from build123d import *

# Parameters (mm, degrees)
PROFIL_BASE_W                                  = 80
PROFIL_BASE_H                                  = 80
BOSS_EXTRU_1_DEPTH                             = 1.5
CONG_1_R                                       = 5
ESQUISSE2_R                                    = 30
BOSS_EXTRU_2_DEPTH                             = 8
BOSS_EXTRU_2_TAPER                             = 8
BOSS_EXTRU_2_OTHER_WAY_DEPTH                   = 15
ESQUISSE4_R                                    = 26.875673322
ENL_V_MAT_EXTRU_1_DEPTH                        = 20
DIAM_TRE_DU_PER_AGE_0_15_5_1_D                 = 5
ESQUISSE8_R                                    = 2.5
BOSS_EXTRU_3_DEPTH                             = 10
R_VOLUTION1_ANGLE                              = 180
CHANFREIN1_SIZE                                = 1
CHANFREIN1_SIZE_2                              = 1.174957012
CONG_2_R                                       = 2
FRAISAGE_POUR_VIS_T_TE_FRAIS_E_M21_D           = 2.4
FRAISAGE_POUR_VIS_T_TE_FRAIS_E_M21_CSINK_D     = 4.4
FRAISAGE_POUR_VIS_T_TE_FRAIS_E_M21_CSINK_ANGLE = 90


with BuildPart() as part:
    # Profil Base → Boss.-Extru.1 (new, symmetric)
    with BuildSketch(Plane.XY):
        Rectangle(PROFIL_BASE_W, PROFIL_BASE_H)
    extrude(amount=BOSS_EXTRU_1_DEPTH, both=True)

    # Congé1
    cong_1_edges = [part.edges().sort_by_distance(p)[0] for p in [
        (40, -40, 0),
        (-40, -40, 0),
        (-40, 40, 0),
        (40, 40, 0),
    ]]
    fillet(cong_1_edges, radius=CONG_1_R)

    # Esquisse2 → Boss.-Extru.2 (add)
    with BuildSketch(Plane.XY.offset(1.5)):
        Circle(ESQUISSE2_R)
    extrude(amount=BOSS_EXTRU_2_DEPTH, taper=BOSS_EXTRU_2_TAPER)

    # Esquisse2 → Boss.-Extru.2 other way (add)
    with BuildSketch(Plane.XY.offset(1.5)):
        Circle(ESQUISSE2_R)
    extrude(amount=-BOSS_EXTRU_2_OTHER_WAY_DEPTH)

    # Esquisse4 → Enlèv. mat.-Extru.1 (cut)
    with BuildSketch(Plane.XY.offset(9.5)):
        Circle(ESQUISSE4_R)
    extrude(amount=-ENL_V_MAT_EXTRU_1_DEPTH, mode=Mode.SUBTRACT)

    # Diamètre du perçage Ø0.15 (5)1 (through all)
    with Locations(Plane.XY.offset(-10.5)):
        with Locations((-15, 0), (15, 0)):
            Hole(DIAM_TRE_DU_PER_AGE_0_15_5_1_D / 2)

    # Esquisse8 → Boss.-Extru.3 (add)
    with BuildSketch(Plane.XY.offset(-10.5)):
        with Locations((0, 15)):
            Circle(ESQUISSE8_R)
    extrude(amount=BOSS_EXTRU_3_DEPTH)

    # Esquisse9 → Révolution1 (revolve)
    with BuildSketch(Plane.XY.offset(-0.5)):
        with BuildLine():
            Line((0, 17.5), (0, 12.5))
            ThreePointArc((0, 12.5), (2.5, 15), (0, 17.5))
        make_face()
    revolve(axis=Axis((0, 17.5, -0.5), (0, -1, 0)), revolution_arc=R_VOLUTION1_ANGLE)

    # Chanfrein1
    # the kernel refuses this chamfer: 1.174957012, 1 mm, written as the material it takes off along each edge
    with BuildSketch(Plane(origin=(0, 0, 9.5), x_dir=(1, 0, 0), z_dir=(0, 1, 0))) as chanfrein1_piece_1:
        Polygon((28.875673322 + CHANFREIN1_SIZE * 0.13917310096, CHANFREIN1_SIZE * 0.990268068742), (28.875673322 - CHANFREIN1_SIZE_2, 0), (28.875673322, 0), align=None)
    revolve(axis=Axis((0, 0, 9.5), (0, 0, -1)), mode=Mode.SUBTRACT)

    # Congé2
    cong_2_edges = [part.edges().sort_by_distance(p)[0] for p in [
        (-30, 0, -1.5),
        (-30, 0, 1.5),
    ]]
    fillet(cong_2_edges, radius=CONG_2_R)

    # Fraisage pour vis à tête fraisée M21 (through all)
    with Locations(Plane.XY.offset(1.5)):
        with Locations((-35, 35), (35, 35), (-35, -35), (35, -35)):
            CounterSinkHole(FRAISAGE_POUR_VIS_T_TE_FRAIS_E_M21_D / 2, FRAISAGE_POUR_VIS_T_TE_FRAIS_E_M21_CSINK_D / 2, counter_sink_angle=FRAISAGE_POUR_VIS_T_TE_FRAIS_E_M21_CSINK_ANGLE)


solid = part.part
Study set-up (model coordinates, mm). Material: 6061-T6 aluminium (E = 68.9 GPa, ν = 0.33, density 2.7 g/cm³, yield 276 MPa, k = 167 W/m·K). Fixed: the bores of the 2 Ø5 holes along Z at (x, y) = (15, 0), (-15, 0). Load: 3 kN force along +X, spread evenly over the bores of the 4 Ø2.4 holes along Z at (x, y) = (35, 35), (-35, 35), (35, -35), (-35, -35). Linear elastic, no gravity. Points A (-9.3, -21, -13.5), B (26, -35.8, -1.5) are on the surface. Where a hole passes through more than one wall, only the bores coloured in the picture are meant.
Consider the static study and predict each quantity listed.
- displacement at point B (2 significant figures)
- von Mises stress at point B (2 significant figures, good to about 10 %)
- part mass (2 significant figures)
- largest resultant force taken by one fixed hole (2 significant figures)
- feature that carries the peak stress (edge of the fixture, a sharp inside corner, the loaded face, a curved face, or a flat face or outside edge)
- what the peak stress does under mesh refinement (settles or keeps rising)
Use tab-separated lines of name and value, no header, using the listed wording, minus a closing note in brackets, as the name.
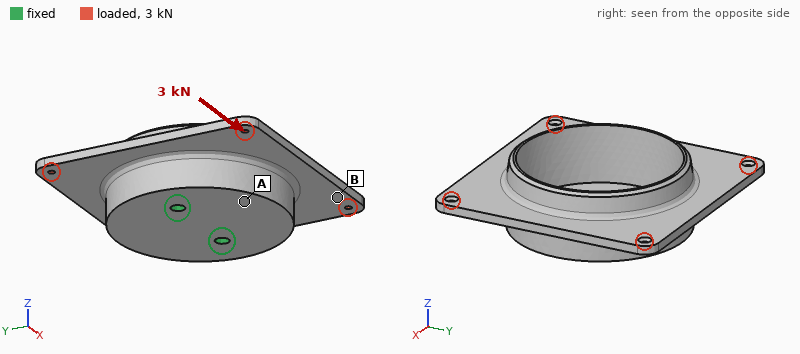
displacement at point B	82 µm
von Mises stress at point B	31 MPa
part mass	80 g
largest resultant force taken by one fixed hole	1.7 kN
feature that carries the peak stress	edge of the fixture
what the peak stress does under mesh refinement	keeps rising
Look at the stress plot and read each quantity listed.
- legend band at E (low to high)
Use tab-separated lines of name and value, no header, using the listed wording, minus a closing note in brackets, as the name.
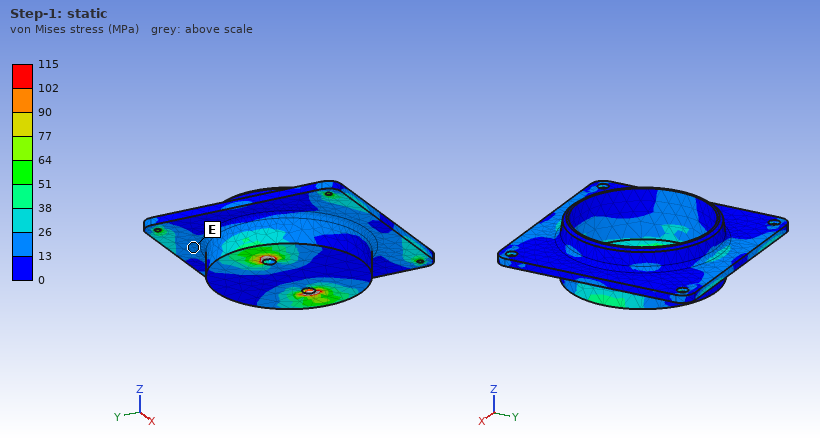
legend band at E	13 to 26 MPa
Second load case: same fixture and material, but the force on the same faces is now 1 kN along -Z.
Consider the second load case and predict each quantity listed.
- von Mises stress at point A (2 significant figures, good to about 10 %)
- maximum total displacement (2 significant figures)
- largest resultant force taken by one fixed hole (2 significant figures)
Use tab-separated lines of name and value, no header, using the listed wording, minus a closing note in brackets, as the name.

von Mises stress at point A	9.6 MPa
maximum total displacement	0.24 mm
largest resultant force taken by one fixed hole	520 N
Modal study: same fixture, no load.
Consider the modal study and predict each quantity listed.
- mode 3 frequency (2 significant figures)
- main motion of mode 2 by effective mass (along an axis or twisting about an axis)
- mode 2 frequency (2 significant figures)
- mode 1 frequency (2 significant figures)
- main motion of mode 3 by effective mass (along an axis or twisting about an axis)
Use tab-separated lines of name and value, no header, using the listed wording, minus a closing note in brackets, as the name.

mode 3 frequency	3600 Hz
main motion of mode 2 by effective mass	along X
mode 2 frequency	2900 Hz
mode 1 frequency	1200 Hz
main motion of mode 3 by effective mass	along Z
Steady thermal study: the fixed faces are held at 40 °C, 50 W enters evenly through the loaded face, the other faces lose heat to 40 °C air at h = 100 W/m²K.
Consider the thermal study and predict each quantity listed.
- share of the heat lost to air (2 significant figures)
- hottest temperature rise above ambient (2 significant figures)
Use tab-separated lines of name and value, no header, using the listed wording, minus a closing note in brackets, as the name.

share of the heat lost to air	52 %
hottest temperature rise above ambient	39 K
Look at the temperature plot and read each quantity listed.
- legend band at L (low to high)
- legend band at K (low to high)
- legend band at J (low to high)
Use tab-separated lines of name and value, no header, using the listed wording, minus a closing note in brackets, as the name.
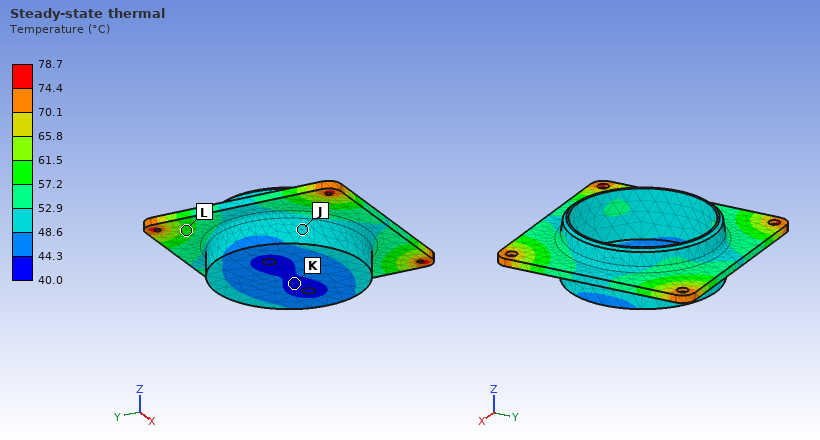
legend band at L	57.2 to 61.5 °C
legend band at K	40.0 to 44.3 °C
legend band at J	48.6 to 52.9 °C
